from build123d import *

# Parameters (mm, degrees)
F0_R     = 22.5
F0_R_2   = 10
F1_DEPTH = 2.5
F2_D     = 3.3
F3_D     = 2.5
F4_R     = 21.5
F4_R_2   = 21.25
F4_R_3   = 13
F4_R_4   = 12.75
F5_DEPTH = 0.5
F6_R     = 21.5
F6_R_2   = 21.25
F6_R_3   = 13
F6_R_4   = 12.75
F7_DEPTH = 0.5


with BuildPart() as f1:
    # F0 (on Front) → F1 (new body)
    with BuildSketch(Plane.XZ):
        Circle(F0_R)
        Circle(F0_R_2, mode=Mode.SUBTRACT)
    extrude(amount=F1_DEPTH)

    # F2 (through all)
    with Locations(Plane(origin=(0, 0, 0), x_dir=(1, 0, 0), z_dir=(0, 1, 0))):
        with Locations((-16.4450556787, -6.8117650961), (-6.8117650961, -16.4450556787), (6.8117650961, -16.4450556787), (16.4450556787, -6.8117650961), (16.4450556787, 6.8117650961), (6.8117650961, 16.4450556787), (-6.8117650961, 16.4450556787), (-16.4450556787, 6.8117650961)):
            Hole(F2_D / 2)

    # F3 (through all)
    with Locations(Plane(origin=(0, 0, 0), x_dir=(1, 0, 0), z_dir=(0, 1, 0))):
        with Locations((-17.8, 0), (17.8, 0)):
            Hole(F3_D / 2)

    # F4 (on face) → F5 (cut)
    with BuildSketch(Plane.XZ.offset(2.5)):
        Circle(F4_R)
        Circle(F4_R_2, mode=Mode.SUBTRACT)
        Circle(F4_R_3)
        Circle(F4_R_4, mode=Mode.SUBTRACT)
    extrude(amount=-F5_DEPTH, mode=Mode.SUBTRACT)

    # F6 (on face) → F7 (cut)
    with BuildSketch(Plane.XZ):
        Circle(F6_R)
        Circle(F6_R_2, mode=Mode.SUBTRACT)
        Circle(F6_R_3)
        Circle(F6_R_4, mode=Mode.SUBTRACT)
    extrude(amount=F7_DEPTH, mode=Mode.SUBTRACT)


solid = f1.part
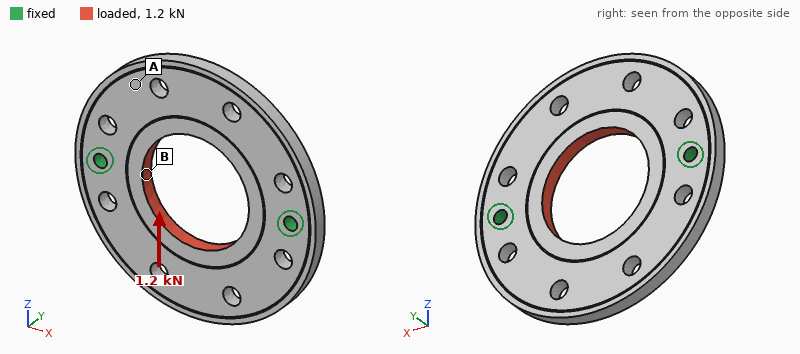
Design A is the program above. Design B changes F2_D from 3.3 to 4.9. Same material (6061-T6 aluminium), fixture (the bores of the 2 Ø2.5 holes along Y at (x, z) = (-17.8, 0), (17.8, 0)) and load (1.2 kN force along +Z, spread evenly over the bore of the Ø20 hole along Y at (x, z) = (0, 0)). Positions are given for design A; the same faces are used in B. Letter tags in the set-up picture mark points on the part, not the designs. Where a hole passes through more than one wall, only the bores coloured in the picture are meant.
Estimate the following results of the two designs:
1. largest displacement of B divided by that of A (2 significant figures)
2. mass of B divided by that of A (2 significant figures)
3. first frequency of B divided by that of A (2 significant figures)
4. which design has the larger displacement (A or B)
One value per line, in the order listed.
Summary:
1.2
0.93
0.97
B
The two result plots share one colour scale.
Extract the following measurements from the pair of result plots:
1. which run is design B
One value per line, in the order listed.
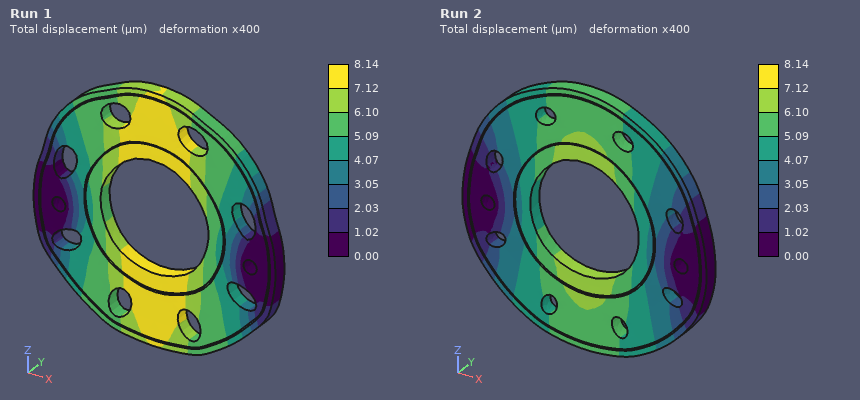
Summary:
Run 1
